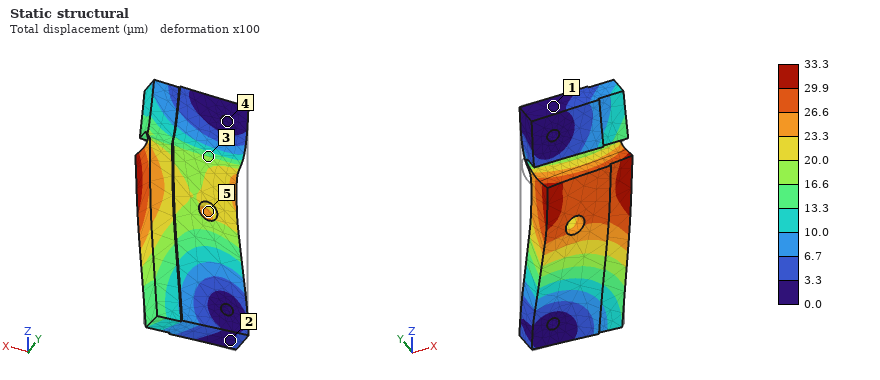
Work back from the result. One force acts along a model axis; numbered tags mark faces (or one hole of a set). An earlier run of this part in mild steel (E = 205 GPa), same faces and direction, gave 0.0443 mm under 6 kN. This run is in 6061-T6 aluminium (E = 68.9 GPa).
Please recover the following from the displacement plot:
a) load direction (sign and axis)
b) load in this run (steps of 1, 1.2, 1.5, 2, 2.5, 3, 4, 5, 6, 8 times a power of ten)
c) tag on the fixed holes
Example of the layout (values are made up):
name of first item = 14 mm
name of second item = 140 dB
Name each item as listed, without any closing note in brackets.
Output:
load direction = +X
load in this run = 1.5 kN
tag on the fixed holes = 4
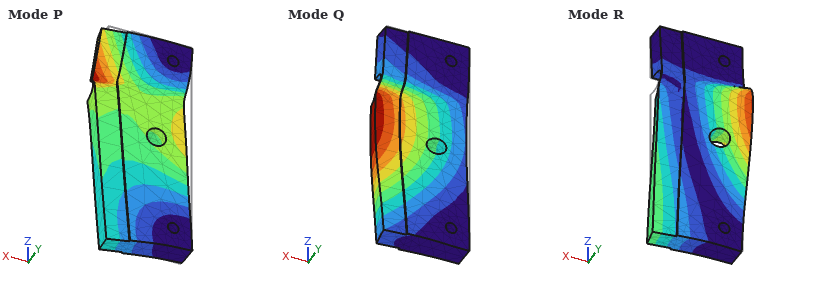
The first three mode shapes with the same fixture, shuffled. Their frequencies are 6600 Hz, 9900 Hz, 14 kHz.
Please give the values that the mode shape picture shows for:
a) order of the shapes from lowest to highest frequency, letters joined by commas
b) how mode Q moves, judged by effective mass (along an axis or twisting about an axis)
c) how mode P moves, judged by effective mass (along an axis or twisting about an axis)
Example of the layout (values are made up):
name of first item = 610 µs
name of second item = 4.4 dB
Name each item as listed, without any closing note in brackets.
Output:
order of the shapes from lowest to highest frequency, letters joined by commas = Q, R, P
how mode Q moves, judged by effective mass = along Y
how mode P moves, judged by effective mass = along X
